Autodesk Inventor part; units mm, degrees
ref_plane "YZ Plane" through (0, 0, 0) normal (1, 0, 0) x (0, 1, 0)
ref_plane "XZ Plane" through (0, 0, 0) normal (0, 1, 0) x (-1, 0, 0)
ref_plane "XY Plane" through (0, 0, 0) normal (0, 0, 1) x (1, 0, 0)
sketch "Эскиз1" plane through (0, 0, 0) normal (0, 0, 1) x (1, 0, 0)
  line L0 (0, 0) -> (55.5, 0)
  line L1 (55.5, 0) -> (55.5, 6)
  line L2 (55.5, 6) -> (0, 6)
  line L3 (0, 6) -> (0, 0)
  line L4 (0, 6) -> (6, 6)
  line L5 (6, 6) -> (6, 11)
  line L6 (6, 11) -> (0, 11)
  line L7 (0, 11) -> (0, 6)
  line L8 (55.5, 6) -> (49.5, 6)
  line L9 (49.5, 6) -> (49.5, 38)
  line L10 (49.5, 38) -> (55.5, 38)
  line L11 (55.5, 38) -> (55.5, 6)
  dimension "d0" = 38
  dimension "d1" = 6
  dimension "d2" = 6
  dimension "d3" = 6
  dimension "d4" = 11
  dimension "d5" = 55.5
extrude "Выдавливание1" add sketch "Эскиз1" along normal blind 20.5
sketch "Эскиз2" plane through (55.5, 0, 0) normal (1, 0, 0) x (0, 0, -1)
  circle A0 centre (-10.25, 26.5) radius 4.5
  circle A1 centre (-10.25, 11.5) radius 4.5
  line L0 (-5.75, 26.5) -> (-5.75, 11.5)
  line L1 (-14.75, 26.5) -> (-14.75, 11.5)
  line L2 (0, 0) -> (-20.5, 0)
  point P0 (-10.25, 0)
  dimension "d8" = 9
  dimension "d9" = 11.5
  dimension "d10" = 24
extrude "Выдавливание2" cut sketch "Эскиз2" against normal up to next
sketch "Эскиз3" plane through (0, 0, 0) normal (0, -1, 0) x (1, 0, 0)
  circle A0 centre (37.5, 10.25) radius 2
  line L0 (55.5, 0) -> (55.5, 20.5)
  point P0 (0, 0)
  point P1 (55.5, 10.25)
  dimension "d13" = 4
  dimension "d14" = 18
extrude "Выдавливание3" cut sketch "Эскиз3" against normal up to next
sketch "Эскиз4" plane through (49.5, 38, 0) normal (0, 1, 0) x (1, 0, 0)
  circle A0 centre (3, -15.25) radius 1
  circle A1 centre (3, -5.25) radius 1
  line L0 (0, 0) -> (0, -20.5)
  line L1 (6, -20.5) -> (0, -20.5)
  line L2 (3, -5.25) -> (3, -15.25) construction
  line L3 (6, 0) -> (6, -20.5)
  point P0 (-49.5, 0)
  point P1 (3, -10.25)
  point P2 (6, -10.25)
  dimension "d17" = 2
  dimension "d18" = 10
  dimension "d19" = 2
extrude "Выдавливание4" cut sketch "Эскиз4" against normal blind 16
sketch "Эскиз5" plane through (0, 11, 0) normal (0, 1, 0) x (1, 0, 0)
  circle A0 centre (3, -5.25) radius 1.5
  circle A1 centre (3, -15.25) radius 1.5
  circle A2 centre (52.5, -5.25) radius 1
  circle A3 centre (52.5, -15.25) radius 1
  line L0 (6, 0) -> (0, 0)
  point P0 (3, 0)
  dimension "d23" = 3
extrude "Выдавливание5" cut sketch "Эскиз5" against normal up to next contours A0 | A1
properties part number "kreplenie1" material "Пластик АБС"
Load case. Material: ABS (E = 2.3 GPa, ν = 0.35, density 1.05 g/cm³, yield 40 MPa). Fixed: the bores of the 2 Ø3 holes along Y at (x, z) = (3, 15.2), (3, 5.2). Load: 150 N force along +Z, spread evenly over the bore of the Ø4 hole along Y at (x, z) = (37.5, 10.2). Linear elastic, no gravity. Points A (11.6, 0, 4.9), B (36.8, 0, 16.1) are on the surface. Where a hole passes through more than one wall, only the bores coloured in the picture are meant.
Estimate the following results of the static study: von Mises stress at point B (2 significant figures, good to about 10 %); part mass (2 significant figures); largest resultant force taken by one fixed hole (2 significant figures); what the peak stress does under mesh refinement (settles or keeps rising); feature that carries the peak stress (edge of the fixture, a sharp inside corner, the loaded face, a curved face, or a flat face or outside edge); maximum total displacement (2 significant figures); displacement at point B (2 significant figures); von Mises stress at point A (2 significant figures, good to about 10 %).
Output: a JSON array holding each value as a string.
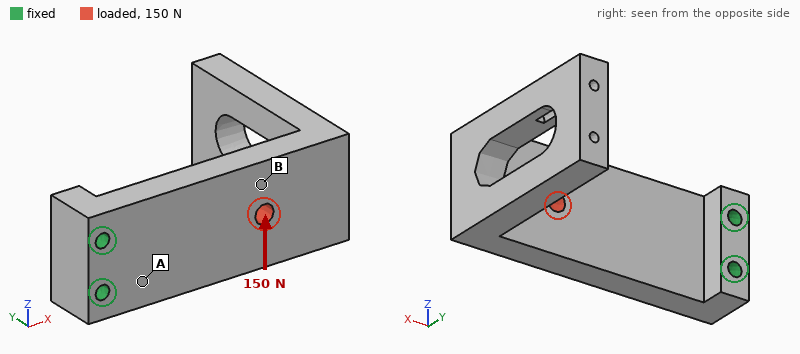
["2.0 MPa", "10 g", "410 N", "keeps rising", "edge of the fixture", "0.52 mm", "0.29 mm", "5.5 MPa"]
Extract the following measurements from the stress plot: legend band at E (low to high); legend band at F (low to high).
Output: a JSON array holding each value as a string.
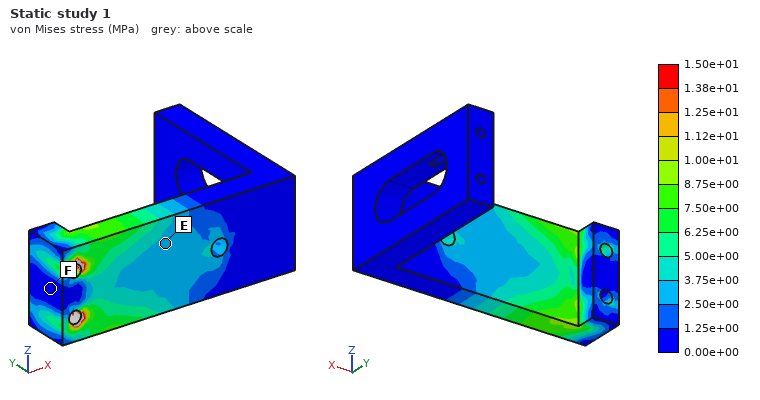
["2.50e+00 to 3.75e+00 MPa", "0.00e+00 to 1.25e+00 MPa"]
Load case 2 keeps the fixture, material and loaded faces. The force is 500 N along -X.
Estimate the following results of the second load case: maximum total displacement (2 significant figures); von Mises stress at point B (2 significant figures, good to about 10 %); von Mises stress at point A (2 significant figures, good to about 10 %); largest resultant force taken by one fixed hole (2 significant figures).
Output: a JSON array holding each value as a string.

["82 µm", "2.3 MPa", "4.3 MPa", "250 N"]
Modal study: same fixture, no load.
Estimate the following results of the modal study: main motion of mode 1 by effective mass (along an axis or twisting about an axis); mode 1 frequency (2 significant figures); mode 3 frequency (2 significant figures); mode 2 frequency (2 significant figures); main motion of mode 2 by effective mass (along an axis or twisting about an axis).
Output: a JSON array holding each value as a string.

["along Y", "300 Hz", "860 Hz", "540 Hz", "along Z"]
